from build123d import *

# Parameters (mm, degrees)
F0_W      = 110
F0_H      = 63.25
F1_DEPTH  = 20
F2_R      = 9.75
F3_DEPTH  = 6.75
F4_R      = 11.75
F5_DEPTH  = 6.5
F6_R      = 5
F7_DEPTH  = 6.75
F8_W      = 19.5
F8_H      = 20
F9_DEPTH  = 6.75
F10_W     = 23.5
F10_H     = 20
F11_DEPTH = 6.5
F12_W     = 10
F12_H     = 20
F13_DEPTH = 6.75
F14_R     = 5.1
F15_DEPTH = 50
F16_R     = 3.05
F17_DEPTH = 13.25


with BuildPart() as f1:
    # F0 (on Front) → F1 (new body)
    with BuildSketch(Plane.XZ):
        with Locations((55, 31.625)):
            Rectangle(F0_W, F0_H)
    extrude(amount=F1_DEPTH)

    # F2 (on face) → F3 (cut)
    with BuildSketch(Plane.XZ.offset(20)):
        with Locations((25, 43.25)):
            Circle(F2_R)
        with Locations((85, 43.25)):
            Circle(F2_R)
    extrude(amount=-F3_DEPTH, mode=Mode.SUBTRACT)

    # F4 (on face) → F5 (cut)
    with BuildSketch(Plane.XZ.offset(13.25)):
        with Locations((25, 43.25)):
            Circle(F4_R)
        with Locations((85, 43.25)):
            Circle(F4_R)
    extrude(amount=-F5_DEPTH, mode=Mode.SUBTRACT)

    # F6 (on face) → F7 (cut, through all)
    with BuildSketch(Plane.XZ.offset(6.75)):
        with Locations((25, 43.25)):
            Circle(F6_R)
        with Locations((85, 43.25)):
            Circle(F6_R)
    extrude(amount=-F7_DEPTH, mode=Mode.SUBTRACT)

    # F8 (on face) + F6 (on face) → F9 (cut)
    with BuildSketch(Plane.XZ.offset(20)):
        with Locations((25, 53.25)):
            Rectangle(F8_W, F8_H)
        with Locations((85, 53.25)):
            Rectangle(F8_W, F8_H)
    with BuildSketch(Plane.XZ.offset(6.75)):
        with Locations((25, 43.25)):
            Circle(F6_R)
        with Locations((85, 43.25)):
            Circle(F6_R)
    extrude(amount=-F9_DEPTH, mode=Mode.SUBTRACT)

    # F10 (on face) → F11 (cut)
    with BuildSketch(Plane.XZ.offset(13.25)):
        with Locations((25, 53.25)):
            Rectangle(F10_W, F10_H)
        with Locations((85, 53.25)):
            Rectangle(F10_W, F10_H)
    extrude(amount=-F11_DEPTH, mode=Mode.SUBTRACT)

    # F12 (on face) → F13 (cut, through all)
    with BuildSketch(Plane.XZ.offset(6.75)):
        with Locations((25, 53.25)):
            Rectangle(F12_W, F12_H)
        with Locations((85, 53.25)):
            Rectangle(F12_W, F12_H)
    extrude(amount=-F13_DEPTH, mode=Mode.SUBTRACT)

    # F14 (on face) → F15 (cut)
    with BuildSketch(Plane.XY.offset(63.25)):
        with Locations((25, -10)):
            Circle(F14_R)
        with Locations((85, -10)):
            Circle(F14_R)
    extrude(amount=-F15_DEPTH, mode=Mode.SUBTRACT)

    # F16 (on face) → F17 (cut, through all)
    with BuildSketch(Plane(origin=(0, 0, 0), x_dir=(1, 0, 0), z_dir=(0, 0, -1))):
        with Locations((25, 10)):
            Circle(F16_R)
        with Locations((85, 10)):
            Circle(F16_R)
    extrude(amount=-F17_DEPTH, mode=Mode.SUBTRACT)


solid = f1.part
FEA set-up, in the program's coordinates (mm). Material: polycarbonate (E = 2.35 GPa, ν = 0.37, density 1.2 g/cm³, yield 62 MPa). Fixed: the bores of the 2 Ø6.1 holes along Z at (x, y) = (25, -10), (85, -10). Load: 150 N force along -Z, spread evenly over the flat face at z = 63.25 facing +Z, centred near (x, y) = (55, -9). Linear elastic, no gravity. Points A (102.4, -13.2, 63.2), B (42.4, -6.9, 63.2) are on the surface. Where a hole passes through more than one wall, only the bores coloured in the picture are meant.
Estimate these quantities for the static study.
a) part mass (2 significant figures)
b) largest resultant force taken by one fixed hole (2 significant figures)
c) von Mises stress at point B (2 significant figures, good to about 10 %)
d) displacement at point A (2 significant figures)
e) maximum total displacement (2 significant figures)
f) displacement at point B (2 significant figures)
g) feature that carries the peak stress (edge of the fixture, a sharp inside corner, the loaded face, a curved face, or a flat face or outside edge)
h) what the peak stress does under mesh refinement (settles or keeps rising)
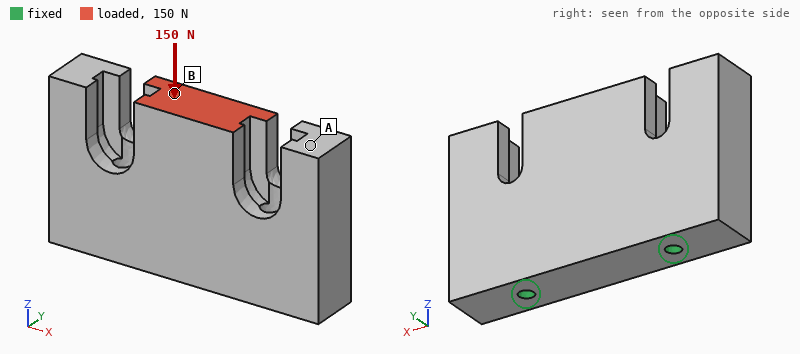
140 g
81 N
0.17 MPa
2.3 µm
6.3 µm
6.1 µm
edge of the fixture
keeps rising
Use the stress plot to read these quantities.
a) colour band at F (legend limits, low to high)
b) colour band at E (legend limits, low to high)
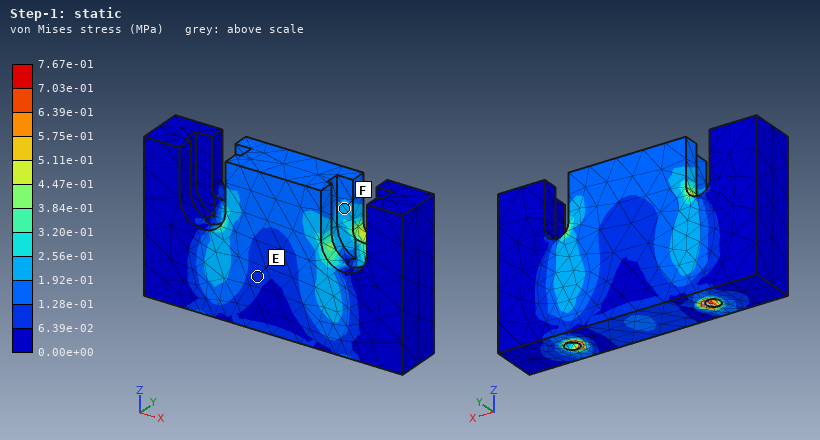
1.92e-01 to 2.56e-01 MPa
6.39e-02 to 1.28e-01 MPa
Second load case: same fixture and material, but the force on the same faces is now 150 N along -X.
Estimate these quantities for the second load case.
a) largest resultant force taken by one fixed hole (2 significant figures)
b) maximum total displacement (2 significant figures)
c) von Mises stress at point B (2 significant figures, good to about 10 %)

150 N
27 µm
0.38 MPa
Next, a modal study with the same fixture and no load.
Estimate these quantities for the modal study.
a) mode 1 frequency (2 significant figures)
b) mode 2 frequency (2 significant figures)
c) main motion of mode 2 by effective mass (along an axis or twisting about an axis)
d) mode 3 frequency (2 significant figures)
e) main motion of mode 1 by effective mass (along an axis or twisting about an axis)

800 Hz
1200 Hz
twisting about Z
1500 Hz
along Y
